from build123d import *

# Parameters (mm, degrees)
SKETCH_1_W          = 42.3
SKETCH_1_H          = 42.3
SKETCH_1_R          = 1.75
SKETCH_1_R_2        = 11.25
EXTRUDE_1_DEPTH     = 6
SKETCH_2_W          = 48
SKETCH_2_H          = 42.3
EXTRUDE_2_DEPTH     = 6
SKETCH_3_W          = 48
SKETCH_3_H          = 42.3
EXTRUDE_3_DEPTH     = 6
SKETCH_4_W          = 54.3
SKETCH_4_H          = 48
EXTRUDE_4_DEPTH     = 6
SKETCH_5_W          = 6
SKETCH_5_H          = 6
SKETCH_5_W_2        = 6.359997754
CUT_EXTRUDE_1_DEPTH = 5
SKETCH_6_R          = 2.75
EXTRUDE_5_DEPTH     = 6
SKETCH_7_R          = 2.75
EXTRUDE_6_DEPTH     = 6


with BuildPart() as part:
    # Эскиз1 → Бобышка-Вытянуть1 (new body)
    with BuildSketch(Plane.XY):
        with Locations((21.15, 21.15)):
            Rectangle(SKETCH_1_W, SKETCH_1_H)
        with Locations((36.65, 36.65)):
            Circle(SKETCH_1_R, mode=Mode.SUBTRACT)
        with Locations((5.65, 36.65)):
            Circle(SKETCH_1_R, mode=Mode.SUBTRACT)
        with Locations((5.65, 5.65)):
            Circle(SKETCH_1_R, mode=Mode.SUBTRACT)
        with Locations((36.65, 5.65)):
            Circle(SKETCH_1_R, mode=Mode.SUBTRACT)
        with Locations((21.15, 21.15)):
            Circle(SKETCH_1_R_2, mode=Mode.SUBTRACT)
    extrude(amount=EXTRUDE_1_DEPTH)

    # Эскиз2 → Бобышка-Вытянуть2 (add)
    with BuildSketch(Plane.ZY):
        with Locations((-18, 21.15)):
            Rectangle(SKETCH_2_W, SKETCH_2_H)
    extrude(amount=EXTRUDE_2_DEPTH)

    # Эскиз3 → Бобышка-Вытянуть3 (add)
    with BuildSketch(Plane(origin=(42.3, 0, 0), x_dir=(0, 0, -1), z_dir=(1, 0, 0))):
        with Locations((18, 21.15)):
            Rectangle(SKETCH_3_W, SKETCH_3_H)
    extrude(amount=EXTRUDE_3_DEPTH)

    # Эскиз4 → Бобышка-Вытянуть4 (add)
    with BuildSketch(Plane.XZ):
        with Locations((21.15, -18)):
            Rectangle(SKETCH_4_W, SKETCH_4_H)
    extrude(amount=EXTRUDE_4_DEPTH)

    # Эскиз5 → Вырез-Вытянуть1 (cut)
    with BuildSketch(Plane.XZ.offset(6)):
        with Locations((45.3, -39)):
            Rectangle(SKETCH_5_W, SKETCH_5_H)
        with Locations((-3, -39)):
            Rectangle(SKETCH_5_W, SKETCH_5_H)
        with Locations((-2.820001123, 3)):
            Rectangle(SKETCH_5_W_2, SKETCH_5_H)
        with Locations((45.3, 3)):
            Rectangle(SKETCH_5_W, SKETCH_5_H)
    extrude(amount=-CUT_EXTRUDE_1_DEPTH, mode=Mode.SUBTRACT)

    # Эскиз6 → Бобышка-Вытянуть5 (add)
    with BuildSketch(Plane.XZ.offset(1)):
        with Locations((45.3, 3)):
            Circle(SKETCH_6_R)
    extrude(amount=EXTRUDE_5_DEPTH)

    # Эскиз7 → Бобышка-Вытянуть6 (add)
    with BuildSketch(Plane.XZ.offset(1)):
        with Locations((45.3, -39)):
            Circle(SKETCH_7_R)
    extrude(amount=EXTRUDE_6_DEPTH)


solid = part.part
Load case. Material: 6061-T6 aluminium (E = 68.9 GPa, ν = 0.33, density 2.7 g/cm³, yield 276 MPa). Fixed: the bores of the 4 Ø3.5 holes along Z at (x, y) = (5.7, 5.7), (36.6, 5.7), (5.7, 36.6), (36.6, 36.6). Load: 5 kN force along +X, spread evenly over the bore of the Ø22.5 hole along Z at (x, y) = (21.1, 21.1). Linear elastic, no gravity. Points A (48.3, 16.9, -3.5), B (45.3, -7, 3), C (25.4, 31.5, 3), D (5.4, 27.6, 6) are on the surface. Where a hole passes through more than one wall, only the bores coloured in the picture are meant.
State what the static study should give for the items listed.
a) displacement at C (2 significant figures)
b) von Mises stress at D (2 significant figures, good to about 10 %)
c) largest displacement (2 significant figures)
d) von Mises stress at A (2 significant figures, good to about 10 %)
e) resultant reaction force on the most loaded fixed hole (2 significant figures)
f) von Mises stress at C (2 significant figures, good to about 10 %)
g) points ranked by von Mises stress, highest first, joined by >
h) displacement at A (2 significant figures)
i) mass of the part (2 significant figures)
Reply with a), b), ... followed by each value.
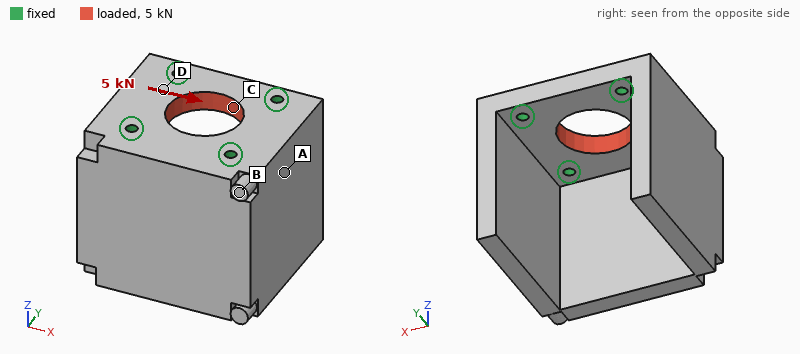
a) 3.0 µm
b) 10.0 MPa
c) 5.0 µm
d) 5.6 MPa
e) 1.3 kN
f) 21 MPa
g) C > D > A > B
h) 2.6 µm
i) 130 g
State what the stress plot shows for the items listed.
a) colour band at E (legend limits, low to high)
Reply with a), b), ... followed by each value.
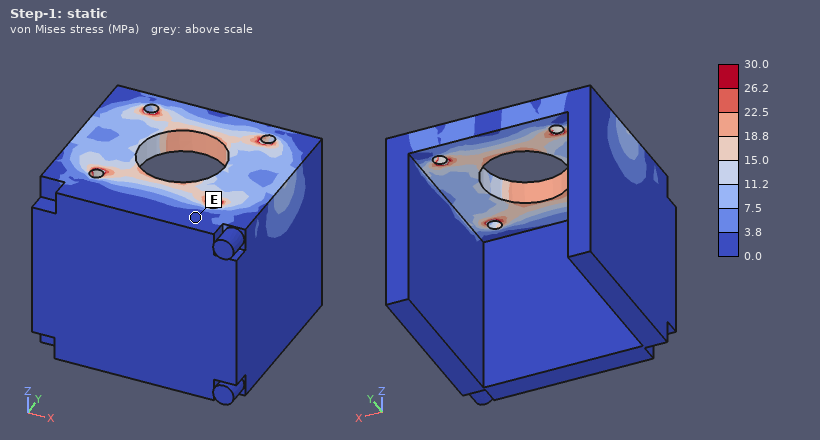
a) 0.0 to 3.8 MPa
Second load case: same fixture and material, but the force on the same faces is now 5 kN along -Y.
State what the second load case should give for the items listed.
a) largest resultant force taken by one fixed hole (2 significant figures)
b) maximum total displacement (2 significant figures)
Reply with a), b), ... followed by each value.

a) 1.3 kN
b) 7.5 µm
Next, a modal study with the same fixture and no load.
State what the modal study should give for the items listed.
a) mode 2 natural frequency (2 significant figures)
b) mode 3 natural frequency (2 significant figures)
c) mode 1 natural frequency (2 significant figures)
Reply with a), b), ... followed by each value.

a) 3400 Hz
b) 5500 Hz
c) 3300 Hz
